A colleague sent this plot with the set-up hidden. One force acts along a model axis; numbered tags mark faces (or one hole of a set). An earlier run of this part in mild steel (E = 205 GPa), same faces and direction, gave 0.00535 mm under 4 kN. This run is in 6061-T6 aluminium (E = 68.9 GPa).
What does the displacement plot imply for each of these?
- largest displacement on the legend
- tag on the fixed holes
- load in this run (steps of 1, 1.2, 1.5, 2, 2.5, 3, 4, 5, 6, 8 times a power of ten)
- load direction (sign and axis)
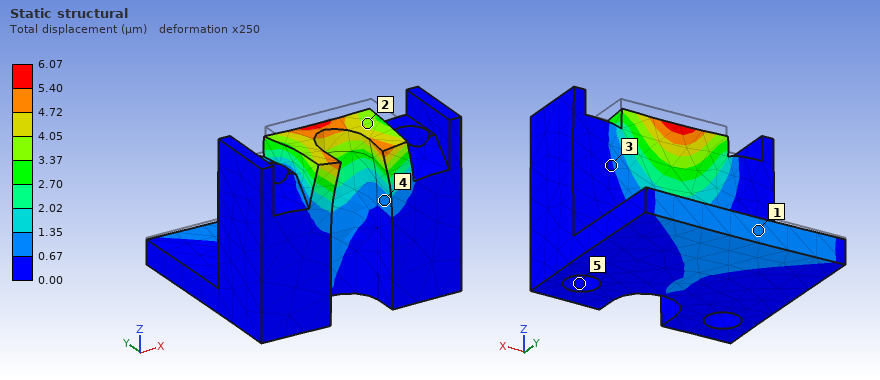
6.07 µm
5
1.5 kN
-Z
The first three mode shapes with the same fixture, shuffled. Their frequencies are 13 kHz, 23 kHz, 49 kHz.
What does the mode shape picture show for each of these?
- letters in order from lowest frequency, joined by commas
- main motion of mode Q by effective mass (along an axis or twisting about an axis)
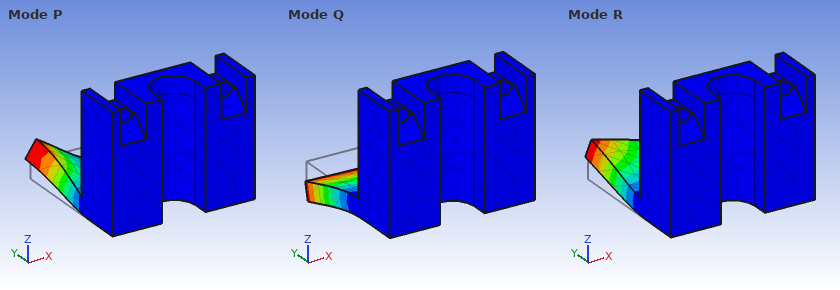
Q, R, P
along Z
